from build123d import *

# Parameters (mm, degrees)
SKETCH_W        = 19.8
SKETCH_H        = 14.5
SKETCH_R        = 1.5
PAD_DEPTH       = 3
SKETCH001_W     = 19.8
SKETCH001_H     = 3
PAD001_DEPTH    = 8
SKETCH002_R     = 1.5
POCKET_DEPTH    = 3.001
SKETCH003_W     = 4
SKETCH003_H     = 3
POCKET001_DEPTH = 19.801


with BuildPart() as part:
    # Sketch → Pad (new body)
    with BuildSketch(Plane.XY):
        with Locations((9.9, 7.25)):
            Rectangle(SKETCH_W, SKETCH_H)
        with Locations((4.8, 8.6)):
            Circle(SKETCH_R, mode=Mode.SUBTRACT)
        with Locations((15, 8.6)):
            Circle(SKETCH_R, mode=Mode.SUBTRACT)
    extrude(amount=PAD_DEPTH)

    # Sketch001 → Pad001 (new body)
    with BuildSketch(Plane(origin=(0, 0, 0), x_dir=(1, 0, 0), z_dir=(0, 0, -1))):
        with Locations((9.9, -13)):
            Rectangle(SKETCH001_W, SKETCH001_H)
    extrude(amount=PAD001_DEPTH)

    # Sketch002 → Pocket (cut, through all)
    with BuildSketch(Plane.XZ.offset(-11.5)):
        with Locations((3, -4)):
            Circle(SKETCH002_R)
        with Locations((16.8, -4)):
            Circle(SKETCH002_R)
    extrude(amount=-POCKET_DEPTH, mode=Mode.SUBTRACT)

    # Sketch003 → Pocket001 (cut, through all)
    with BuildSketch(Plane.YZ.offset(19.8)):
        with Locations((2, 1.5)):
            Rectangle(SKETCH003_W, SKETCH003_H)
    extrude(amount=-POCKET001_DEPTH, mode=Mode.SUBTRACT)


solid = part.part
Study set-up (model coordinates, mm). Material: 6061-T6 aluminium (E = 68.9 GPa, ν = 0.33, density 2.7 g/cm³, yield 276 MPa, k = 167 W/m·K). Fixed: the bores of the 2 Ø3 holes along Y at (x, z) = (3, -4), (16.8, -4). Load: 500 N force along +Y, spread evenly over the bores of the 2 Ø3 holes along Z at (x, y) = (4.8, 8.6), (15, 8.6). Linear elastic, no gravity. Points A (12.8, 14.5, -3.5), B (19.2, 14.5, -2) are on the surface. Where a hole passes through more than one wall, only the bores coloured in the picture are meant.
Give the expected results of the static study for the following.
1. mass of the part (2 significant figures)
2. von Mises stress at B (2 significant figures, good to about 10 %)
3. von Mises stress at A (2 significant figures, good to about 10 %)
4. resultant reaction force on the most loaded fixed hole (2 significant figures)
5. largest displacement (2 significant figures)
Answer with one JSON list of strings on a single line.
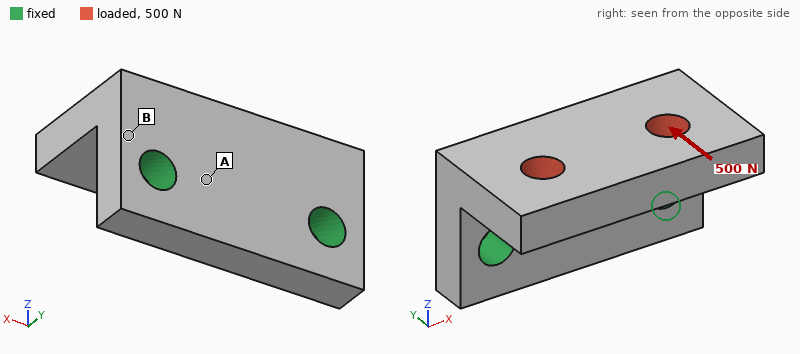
["2.7 g", "56 MPa", "26 MPa", "250 N", "24 µm"]
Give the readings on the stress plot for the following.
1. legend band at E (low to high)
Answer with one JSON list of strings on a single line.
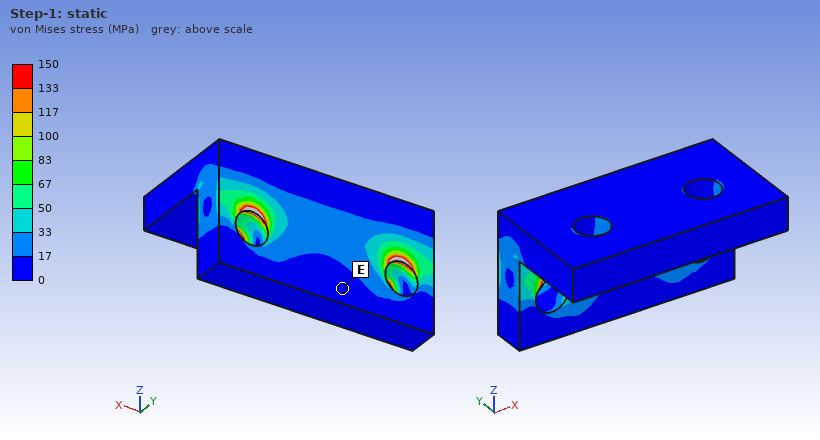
["0 to 17 MPa"]
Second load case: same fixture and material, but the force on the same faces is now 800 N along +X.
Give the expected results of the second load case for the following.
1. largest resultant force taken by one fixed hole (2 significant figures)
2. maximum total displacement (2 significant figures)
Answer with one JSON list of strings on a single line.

["530 N", "17 µm"]
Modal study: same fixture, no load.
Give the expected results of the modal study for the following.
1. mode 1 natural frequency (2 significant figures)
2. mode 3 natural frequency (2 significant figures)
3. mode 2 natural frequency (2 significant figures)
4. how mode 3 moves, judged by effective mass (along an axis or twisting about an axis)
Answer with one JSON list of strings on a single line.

["16 kHz", "39 kHz", "27 kHz", "along X"]
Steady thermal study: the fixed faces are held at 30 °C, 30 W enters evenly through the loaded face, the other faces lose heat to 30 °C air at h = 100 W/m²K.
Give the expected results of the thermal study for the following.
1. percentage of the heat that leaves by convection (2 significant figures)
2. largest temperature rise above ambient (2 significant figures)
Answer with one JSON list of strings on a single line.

["4.2 %", "31 K"]
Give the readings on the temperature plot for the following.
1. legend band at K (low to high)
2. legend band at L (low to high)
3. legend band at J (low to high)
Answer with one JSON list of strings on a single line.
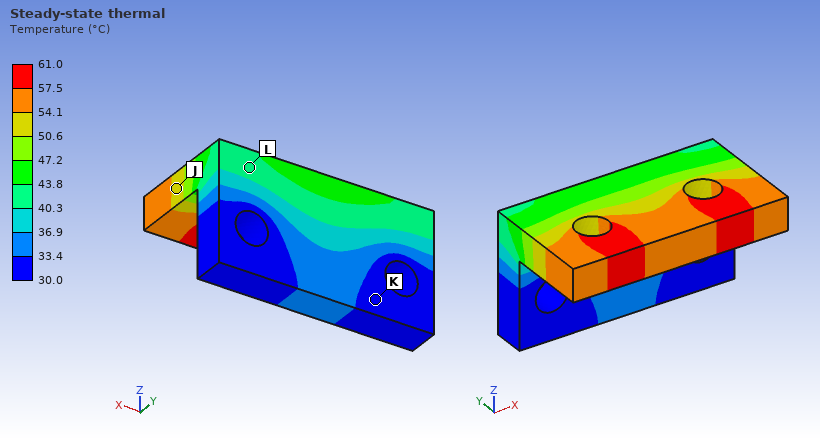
["30.0 to 33.4 °C", "40.3 to 43.8 °C", "50.6 to 54.1 °C"]
